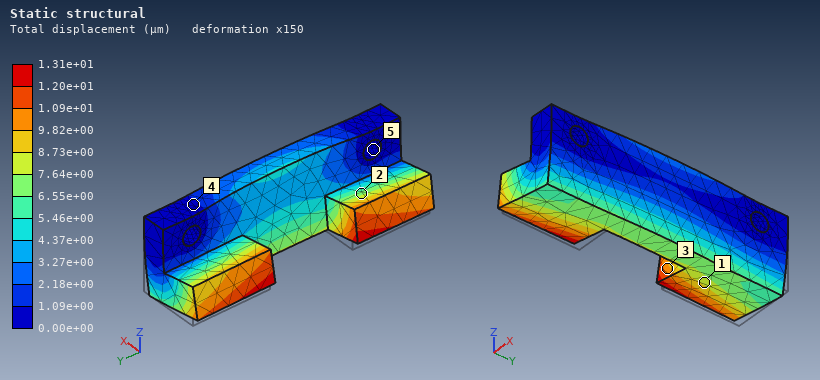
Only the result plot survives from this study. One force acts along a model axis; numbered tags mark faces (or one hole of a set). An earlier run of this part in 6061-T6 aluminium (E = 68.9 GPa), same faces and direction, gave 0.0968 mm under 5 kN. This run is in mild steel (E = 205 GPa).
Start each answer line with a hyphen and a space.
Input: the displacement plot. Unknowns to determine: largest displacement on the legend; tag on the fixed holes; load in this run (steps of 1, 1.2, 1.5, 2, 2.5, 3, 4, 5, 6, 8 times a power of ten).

- 1.31e+01 µm
- 5
- 2 kN
